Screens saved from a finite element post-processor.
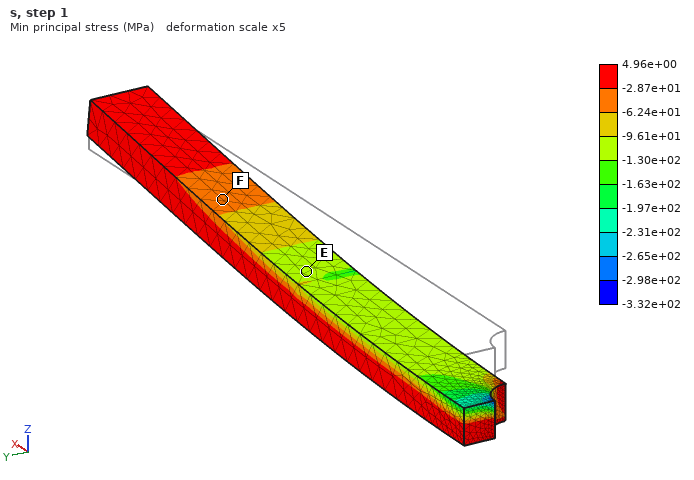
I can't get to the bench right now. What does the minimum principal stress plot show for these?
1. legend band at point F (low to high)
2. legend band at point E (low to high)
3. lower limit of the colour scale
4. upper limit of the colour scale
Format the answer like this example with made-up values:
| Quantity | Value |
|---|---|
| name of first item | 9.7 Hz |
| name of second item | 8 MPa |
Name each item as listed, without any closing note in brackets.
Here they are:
| Quantity | Value |
|---|---|
| legend band at point F | -6.24e+01 to -2.87e+01 MPa |
| legend band at point E | -1.30e+02 to -9.61e+01 MPa |
| lower limit of the colour scale | -3.32e+02 MPa |
| upper limit of the colour scale | 4.96e+00 MPa |
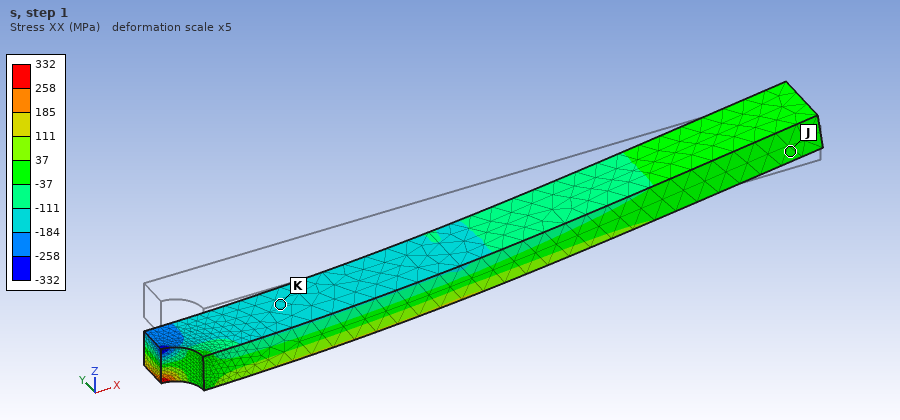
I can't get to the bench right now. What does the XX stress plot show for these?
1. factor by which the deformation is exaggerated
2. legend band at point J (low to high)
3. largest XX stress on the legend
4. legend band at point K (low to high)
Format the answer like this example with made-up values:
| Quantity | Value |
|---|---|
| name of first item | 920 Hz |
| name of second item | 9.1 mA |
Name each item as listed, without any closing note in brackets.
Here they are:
| Quantity | Value |
|---|---|
| factor by which the deformation is exaggerated | 5 |
| legend band at point J | -37 to 37 MPa |
| largest XX stress on the legend | 332 MPa |
| legend band at point K | -184 to -111 MPa |
